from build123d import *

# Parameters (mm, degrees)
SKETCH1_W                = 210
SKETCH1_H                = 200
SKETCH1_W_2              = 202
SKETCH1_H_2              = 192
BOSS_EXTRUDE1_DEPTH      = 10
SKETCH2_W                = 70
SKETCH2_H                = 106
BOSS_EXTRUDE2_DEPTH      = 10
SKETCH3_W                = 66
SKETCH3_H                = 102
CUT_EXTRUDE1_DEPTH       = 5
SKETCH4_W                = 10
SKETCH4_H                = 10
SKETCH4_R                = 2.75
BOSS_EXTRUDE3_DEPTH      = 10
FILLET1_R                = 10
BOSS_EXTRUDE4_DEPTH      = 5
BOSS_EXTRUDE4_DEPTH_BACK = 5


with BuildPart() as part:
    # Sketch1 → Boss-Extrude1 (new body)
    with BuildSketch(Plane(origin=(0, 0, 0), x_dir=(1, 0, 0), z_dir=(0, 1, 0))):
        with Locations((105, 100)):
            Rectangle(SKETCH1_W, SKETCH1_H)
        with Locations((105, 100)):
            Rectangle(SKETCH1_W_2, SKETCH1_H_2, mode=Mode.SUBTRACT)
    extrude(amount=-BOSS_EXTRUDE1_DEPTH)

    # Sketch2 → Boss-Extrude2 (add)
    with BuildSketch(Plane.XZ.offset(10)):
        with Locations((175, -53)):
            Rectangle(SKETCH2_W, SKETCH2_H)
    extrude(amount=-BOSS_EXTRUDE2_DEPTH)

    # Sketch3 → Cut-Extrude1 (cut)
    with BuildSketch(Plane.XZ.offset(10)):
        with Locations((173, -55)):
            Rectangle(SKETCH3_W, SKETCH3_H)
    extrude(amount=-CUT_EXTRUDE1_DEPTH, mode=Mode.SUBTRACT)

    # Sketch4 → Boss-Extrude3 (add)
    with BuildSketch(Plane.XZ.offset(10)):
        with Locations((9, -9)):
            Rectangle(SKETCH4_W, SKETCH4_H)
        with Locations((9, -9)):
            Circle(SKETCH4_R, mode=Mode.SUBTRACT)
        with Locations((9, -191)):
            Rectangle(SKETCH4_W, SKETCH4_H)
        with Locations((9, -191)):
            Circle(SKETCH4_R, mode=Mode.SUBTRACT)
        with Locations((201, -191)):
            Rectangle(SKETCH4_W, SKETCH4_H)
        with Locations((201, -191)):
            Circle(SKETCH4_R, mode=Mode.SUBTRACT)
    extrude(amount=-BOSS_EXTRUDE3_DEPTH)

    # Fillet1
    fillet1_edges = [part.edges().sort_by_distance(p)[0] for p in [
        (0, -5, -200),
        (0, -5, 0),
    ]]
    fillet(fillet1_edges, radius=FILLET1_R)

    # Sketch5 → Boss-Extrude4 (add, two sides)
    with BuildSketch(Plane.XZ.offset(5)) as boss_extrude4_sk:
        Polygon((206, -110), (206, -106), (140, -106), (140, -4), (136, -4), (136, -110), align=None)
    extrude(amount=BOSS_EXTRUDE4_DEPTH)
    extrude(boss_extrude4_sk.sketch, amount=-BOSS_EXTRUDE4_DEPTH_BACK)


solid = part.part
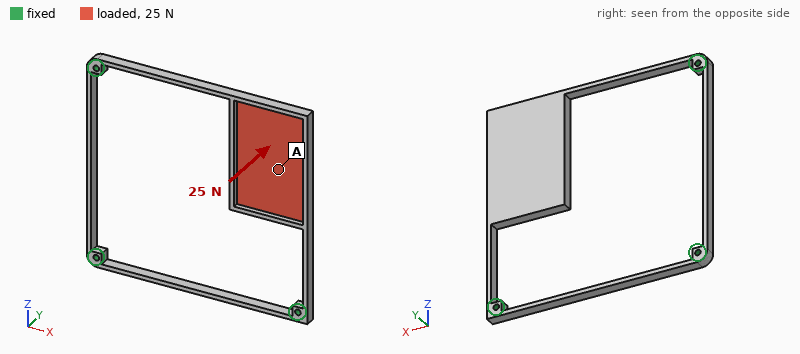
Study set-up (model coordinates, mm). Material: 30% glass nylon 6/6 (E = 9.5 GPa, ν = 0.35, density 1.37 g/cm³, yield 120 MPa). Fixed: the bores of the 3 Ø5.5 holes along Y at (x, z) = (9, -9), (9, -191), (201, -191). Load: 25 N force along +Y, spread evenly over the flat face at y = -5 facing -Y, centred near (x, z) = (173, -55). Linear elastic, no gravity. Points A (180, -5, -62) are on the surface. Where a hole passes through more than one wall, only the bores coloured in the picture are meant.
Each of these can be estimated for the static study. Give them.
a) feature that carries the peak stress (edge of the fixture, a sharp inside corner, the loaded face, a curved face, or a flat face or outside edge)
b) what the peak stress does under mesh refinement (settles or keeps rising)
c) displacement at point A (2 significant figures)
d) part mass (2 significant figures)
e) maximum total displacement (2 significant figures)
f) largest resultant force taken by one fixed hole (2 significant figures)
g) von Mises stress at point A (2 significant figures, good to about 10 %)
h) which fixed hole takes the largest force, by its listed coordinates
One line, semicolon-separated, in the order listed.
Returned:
a sharp inside corner; keeps rising; 1.5 mm; 100 g; 3.1 mm; 14 N; 1.5 MPa; (201, -191)
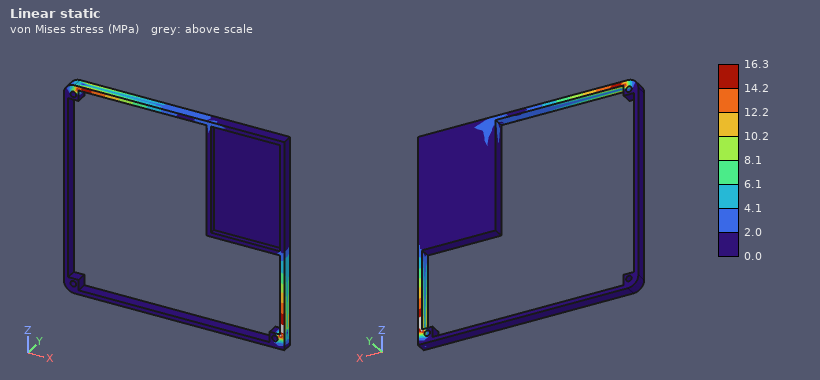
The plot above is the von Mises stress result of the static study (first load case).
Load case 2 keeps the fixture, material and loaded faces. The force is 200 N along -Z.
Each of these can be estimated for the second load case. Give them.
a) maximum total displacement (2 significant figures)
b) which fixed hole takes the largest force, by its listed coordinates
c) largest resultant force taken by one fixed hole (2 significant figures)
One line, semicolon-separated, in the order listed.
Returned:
3.0 mm; (201, -191); 200 N
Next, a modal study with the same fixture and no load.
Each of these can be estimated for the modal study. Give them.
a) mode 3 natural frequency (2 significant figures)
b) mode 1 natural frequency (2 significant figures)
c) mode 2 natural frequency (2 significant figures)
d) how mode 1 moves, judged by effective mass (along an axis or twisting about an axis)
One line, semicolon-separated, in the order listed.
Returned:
190 Hz; 70 Hz; 140 Hz; along Y
